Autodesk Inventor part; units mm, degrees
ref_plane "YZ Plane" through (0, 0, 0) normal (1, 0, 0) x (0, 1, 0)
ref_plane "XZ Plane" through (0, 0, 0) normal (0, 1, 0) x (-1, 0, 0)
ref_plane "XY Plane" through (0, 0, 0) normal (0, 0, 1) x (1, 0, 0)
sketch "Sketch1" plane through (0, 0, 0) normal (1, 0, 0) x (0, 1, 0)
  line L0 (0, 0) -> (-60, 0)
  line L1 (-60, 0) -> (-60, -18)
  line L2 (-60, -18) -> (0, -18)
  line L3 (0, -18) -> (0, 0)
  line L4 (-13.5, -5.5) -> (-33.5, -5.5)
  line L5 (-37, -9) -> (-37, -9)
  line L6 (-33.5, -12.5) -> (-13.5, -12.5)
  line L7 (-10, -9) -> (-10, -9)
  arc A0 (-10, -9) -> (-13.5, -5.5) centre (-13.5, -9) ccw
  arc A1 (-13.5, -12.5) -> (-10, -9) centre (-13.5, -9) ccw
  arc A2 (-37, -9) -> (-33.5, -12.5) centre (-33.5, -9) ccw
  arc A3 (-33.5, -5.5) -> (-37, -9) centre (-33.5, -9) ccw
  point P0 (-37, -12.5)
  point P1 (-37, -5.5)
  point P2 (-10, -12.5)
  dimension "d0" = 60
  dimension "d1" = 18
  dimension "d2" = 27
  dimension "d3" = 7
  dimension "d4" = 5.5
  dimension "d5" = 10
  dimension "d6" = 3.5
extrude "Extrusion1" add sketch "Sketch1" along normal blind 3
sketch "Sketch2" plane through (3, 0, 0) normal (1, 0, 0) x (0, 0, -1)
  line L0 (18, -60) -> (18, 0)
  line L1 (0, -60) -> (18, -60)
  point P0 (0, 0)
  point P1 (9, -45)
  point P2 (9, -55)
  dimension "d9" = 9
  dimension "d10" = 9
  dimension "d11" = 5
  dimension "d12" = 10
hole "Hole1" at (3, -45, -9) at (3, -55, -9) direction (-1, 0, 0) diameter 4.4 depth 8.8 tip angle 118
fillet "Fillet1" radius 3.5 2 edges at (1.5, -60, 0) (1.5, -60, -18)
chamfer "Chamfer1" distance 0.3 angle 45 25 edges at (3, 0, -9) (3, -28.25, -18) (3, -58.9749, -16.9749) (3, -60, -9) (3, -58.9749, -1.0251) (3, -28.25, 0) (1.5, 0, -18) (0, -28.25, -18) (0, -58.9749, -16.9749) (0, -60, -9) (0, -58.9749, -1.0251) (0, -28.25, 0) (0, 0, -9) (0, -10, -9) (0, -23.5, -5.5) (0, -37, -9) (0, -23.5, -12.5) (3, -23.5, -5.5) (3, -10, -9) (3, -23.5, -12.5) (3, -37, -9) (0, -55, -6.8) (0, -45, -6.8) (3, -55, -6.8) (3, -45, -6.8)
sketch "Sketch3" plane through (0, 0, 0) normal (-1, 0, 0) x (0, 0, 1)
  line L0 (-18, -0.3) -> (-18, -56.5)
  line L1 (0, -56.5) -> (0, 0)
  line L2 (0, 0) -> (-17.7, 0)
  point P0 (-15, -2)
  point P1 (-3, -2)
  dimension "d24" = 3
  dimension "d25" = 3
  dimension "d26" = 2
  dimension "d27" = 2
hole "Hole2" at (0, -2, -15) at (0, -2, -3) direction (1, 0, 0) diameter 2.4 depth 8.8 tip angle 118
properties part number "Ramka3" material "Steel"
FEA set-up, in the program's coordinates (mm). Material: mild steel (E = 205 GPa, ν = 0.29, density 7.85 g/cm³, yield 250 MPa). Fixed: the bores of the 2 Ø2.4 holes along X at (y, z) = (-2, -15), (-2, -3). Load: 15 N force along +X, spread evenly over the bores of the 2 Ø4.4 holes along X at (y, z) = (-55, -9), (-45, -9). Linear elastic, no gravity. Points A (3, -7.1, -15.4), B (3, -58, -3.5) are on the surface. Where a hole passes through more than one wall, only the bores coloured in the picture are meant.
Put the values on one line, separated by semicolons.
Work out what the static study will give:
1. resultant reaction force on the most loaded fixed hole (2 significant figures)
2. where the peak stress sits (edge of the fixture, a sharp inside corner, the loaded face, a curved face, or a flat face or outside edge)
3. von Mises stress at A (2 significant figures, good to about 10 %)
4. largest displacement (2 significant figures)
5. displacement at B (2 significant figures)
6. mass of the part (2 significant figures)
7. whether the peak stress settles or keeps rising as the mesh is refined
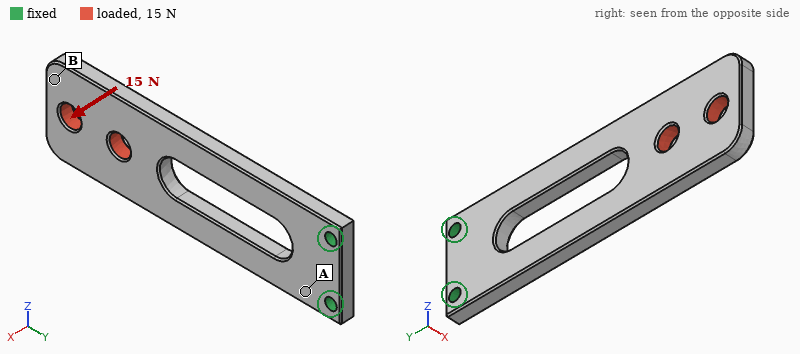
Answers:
7.5 N; edge of the fixture; 27 MPa; 0.12 mm; 0.12 mm; 20 g; keeps rising
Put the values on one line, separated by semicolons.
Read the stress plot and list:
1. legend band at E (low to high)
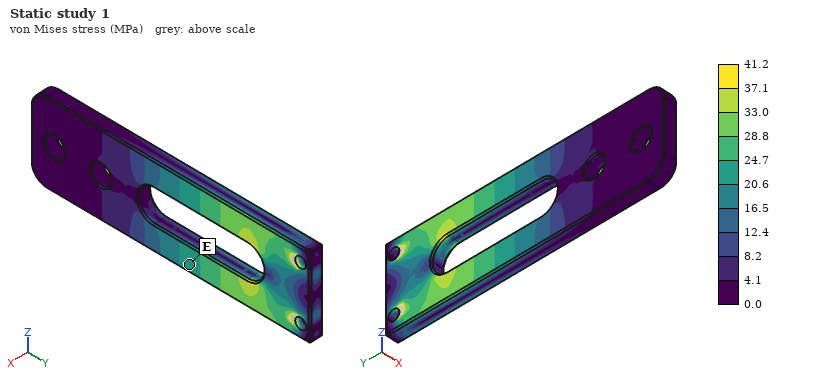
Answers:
20.6 to 24.7 MPa
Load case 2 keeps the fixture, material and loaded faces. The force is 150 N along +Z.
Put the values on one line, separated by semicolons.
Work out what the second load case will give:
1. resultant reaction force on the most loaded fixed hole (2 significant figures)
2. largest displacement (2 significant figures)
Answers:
550 N; 46 µm
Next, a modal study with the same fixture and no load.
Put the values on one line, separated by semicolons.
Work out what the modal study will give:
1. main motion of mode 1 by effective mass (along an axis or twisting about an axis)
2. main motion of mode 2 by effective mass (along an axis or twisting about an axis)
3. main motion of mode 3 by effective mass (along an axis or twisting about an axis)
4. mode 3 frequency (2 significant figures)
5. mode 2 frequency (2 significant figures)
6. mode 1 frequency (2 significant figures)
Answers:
along X; along Z; twisting about Y; 3600 Hz; 3100 Hz; 670 Hz
